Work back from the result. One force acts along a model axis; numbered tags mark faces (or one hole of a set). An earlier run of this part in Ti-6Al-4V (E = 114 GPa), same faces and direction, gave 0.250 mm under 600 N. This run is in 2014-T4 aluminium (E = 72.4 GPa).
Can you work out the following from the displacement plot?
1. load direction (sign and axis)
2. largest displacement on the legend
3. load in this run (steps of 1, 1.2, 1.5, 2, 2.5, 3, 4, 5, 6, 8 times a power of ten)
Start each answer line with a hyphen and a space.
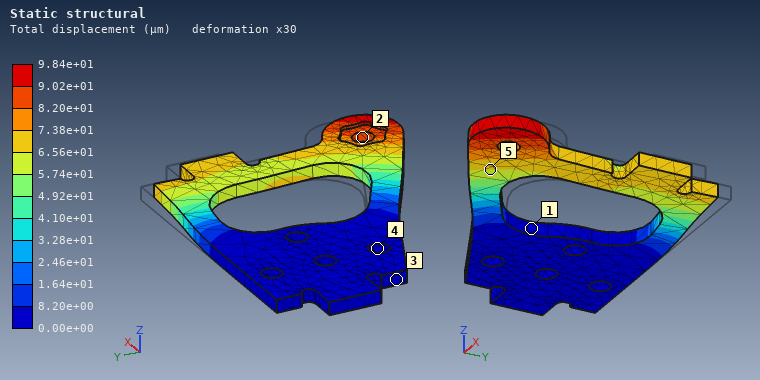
- -Y
- 9.84e+01 µm
- 150 N
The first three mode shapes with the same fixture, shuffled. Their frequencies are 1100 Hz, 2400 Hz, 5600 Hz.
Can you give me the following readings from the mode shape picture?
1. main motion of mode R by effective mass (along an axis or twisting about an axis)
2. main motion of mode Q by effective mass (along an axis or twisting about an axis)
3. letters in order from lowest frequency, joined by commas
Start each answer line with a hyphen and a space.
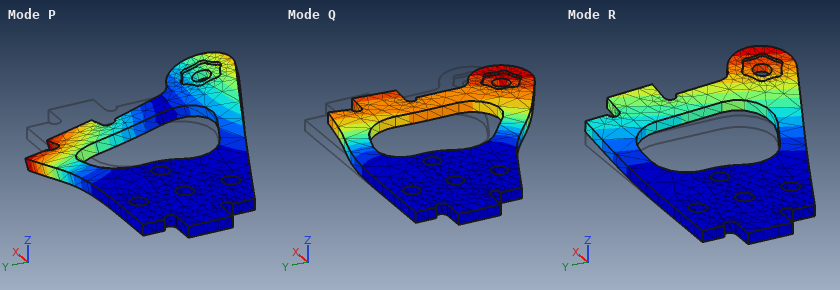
- along Z
- along Y
- R, P, Q
